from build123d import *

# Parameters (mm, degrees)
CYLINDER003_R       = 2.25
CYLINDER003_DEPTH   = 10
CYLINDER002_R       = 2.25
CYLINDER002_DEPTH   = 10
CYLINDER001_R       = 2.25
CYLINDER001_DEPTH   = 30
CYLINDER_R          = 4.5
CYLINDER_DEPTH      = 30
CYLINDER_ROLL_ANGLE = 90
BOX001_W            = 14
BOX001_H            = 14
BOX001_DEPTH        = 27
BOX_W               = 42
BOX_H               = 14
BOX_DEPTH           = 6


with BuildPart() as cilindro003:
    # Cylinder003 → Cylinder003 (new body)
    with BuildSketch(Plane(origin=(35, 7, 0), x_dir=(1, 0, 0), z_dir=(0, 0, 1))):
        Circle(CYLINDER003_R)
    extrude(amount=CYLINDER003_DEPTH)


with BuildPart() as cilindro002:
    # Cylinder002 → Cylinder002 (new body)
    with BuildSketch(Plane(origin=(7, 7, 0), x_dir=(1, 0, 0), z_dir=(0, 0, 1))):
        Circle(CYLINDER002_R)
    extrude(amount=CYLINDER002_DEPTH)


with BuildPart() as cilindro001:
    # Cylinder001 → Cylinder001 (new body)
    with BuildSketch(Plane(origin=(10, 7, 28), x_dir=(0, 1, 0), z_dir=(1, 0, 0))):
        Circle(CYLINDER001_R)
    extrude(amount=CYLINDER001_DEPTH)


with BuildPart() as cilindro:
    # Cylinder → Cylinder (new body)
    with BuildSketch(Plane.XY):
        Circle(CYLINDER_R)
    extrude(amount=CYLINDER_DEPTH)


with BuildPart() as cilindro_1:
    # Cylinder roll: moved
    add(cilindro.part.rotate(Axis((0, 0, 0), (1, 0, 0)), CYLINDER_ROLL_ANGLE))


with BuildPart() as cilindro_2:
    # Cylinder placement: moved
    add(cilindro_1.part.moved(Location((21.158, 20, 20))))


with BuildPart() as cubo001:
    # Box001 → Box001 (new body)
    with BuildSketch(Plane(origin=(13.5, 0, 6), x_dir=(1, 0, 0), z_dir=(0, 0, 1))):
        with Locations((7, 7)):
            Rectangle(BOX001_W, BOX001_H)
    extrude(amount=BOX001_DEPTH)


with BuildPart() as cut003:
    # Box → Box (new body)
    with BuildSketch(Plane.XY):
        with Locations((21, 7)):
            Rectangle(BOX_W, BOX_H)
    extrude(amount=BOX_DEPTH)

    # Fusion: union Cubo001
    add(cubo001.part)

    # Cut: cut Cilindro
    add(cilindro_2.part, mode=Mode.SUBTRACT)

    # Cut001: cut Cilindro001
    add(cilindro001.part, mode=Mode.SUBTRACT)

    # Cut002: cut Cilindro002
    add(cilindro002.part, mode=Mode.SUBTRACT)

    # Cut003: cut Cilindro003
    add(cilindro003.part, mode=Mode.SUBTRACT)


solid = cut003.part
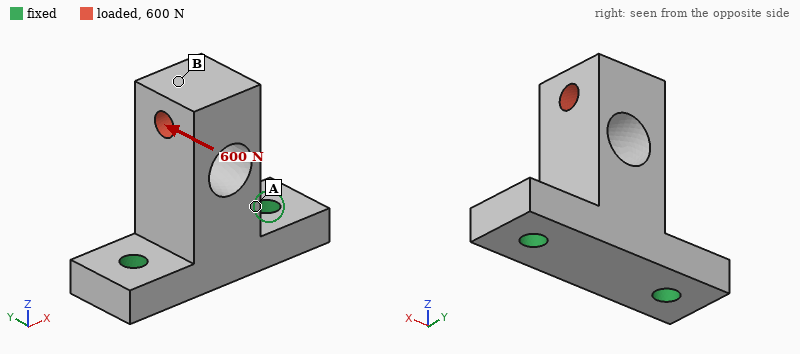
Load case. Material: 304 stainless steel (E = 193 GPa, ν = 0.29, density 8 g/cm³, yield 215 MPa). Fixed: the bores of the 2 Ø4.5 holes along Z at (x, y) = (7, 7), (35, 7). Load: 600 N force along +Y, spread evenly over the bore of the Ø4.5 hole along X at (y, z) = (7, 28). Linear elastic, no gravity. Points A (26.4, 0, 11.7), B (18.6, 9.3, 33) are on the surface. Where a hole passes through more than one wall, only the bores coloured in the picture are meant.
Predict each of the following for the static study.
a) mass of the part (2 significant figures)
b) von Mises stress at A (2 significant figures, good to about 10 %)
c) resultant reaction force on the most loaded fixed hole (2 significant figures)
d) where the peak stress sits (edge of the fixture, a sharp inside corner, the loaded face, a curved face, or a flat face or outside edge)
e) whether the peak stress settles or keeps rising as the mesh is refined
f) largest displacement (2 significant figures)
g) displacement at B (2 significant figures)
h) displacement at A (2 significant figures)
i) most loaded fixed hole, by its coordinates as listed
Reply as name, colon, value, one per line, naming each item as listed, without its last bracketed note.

mass of the part: 60 g
von Mises stress at A: 28 MPa
resultant reaction force on the most loaded fixed hole: 320 N
where the peak stress sits: edge of the fixture
whether the peak stress settles or keeps rising as the mesh is refined: keeps rising
largest displacement: 38 µm
displacement at B: 37 µm
displacement at A: 12 µm
most loaded fixed hole, by its coordinates as listed: (7, 7)
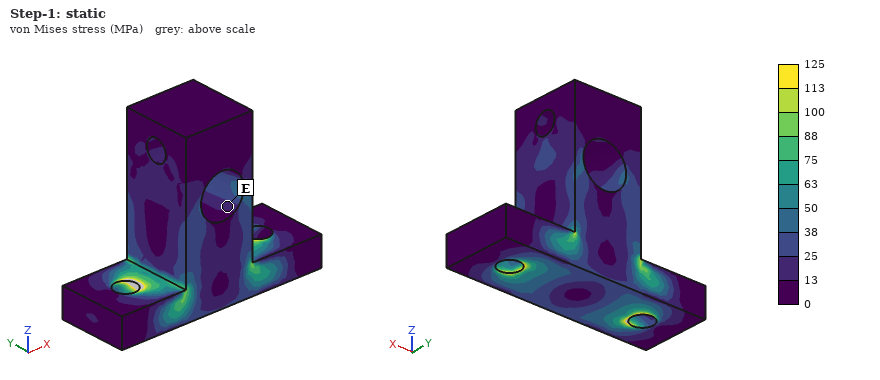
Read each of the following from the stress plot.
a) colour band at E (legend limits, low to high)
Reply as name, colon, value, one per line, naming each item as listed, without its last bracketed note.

colour band at E: 13 to 25 MPa
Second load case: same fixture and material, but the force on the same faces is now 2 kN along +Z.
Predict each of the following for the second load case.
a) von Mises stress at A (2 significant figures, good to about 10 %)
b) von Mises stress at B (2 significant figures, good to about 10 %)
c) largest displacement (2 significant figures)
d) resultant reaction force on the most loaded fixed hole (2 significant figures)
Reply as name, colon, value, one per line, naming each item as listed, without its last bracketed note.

von Mises stress at A: 20 MPa
von Mises stress at B: 9.8 MPa
largest displacement: 6.5 µm
resultant reaction force on the most loaded fixed hole: 1.1 kN
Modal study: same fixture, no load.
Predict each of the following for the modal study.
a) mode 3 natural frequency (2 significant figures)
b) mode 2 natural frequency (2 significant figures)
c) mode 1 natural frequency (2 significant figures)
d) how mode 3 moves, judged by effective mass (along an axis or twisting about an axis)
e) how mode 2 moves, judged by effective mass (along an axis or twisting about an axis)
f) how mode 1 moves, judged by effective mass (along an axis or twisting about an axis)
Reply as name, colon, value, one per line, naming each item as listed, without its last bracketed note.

mode 3 natural frequency: 19 kHz
mode 2 natural frequency: 8400 Hz
mode 1 natural frequency: 5300 Hz
how mode 3 moves, judged by effective mass: along Z
how mode 2 moves, judged by effective mass: along X
how mode 1 moves, judged by effective mass: along Y
